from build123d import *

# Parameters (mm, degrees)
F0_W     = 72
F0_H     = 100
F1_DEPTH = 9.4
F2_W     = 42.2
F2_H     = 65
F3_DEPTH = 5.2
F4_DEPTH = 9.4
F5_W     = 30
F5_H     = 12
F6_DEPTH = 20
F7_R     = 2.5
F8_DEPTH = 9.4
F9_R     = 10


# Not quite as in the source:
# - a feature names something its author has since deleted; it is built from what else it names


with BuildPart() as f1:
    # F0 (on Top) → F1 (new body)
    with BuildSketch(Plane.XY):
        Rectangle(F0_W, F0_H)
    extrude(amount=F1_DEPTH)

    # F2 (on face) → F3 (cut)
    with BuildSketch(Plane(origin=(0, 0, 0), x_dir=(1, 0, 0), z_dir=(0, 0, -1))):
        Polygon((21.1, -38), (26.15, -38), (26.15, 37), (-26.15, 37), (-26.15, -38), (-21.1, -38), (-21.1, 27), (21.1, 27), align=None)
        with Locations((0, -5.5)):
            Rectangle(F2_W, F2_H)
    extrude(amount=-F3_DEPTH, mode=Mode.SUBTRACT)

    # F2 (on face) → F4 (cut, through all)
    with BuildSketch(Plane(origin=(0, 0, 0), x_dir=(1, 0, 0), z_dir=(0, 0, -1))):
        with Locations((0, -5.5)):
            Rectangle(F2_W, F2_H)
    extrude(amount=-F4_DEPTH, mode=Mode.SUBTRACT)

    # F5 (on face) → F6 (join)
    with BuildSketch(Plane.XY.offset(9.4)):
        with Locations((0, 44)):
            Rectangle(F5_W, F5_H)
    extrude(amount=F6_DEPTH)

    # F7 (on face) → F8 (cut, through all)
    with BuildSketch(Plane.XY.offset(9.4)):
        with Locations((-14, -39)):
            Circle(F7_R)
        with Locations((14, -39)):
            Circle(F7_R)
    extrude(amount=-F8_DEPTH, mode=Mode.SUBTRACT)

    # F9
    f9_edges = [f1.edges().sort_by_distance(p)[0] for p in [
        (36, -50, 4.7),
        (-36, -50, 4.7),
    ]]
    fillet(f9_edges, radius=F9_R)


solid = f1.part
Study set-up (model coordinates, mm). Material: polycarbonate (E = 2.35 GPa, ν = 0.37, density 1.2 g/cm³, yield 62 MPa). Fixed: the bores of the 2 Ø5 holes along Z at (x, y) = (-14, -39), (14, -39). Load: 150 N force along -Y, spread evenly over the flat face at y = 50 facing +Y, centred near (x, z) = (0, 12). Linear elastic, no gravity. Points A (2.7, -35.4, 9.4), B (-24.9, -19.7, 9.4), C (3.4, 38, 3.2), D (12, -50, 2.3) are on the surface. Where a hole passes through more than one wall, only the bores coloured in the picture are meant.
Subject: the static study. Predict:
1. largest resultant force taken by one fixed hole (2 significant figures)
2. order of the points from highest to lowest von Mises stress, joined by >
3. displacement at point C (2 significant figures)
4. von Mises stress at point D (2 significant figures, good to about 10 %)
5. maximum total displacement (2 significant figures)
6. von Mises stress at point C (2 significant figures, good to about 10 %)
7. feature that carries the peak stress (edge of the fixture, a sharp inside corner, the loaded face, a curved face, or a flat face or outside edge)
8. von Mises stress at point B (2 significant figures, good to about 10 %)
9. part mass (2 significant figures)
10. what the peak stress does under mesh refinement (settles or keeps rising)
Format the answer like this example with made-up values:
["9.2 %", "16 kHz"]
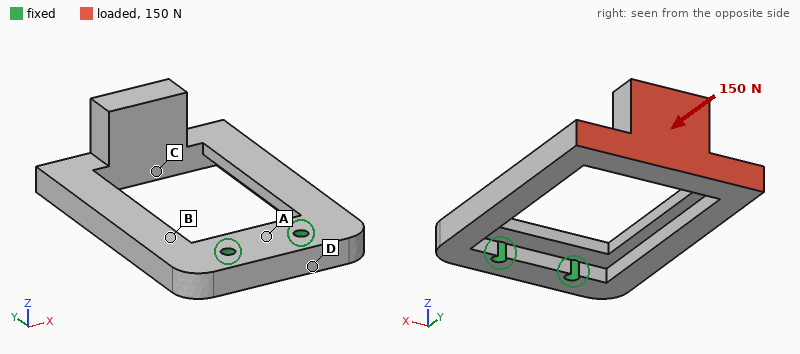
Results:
["76 N", "B > C > D > A", "0.84 mm", "1.1 MPa", "1.4 mm", "1.7 MPa", "edge of the fixture", "3.4 MPa", "51 g", "keeps rising"]
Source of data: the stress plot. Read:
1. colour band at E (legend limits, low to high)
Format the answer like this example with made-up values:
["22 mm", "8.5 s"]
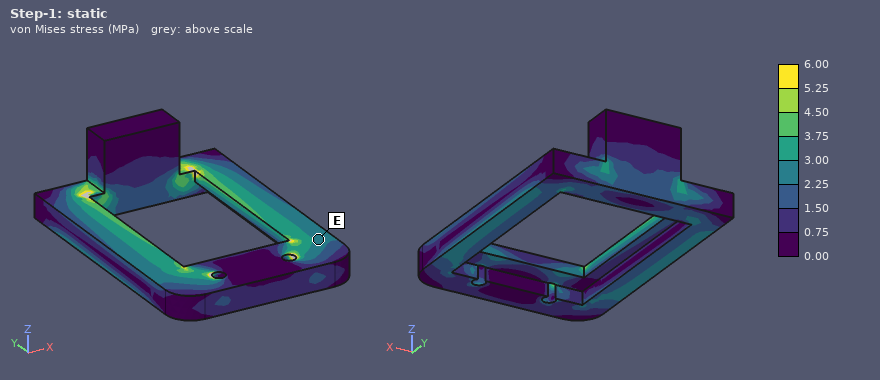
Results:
["2.25 to 3.00 MPa"]
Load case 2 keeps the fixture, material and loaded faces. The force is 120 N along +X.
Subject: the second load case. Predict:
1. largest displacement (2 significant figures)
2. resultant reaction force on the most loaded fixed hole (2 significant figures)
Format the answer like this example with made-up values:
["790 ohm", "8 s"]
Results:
["1.3 mm", "290 N"]
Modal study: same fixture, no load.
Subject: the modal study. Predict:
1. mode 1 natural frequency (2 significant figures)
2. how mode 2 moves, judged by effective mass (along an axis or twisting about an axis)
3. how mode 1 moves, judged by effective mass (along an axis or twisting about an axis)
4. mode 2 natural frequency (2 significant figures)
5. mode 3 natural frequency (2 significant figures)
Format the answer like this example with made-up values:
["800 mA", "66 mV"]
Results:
["130 Hz", "along X", "along Z", "320 Hz", "340 Hz"]
